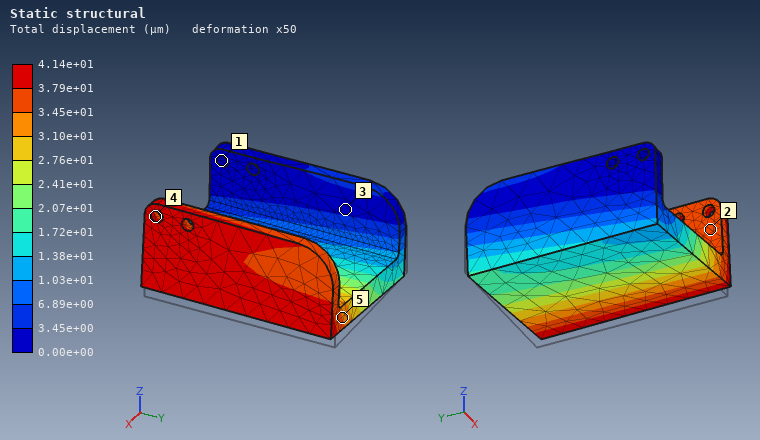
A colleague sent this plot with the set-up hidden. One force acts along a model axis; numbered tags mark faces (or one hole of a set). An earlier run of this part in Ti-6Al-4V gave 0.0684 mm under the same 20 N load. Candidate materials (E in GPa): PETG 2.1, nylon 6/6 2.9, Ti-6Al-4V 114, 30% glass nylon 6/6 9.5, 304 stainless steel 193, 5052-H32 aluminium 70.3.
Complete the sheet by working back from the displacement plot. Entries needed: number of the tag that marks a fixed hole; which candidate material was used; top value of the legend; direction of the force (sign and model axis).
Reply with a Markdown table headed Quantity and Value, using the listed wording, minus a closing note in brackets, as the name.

| Quantity | Value |
|---|---|
| number of the tag that marks a fixed hole | 1 |
| which candidate material was used | 304 stainless steel |
| top value of the legend | 4.14e+01 µm |
| direction of the force | +Z |
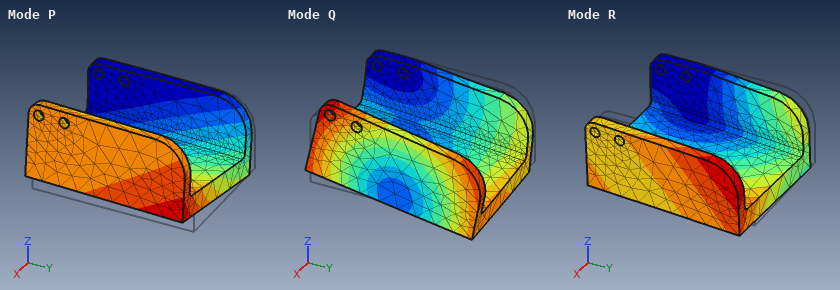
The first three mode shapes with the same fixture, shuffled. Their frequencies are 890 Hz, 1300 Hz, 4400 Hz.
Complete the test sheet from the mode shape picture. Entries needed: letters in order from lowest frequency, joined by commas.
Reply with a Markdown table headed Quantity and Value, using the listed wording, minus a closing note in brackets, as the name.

| Quantity | Value |
|---|---|
| letters in order from lowest frequency, joined by commas | P, R, Q |
